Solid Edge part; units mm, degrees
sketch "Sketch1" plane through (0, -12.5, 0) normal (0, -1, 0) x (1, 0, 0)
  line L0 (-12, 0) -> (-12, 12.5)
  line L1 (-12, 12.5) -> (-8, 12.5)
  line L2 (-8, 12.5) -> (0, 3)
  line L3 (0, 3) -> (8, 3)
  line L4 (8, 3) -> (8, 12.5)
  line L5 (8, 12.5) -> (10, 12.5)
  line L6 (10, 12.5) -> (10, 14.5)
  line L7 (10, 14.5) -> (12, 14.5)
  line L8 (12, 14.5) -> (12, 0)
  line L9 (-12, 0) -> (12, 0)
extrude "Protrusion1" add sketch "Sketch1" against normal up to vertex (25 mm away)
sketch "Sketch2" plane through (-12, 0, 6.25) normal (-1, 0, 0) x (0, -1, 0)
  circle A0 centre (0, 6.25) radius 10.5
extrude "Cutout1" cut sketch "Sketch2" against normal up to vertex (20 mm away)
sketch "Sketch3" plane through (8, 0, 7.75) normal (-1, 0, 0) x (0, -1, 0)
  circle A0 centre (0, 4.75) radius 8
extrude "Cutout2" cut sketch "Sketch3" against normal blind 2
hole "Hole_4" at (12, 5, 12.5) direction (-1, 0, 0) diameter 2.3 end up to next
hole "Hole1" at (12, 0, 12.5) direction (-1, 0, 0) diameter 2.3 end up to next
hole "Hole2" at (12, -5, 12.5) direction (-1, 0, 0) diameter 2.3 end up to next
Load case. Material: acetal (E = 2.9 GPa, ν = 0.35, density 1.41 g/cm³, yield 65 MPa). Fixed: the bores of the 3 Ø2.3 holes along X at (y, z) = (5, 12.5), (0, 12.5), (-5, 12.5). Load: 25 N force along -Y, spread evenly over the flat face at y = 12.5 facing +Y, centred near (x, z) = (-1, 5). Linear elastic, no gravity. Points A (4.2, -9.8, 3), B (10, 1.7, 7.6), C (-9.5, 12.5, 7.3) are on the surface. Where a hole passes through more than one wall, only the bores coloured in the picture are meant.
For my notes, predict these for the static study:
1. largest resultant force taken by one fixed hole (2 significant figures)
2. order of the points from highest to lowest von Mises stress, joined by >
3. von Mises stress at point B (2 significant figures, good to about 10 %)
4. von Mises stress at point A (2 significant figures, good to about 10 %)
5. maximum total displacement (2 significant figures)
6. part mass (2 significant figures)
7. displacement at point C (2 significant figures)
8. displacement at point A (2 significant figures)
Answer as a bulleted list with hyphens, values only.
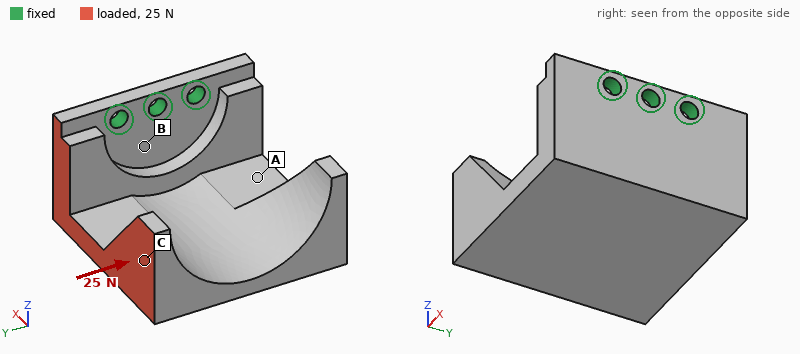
- 27 N
- B > A > C
- 5.7 MPa
- 3.0 MPa
- 0.40 mm
- 4.4 g
- 0.33 mm
- 0.14 mm
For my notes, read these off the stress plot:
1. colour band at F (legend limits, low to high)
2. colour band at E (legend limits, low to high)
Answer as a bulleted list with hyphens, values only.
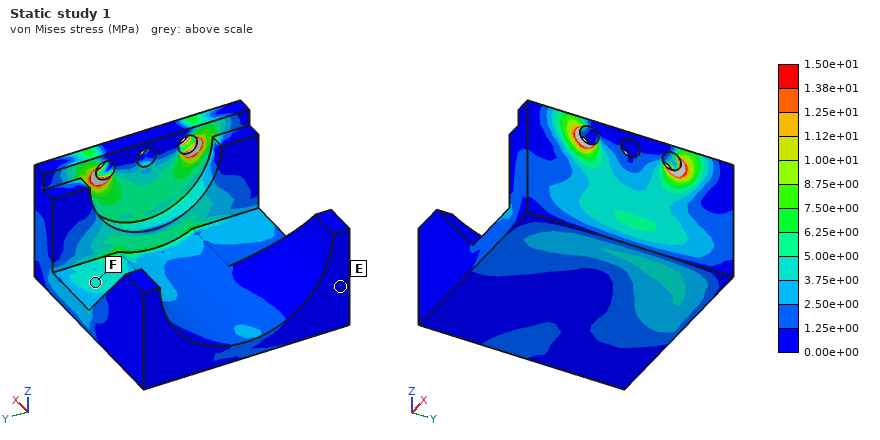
- 3.75e+00 to 5.00e+00 MPa
- 0.00e+00 to 1.25e+00 MPa
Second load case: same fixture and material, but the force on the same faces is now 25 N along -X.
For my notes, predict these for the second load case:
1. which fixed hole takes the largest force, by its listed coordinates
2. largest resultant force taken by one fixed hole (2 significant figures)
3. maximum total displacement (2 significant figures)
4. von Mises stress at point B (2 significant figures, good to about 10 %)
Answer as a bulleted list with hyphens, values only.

- (5, 12.5)
- 31 N
- 0.38 mm
- 5.2 MPa
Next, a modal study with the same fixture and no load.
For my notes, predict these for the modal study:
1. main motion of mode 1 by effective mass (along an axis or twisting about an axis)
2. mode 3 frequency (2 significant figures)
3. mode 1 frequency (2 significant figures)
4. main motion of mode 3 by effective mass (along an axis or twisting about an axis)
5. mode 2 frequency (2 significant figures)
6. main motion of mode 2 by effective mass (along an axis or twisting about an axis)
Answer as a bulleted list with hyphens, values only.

- along Z
- 1800 Hz
- 520 Hz
- along X
- 820 Hz
- along Y
